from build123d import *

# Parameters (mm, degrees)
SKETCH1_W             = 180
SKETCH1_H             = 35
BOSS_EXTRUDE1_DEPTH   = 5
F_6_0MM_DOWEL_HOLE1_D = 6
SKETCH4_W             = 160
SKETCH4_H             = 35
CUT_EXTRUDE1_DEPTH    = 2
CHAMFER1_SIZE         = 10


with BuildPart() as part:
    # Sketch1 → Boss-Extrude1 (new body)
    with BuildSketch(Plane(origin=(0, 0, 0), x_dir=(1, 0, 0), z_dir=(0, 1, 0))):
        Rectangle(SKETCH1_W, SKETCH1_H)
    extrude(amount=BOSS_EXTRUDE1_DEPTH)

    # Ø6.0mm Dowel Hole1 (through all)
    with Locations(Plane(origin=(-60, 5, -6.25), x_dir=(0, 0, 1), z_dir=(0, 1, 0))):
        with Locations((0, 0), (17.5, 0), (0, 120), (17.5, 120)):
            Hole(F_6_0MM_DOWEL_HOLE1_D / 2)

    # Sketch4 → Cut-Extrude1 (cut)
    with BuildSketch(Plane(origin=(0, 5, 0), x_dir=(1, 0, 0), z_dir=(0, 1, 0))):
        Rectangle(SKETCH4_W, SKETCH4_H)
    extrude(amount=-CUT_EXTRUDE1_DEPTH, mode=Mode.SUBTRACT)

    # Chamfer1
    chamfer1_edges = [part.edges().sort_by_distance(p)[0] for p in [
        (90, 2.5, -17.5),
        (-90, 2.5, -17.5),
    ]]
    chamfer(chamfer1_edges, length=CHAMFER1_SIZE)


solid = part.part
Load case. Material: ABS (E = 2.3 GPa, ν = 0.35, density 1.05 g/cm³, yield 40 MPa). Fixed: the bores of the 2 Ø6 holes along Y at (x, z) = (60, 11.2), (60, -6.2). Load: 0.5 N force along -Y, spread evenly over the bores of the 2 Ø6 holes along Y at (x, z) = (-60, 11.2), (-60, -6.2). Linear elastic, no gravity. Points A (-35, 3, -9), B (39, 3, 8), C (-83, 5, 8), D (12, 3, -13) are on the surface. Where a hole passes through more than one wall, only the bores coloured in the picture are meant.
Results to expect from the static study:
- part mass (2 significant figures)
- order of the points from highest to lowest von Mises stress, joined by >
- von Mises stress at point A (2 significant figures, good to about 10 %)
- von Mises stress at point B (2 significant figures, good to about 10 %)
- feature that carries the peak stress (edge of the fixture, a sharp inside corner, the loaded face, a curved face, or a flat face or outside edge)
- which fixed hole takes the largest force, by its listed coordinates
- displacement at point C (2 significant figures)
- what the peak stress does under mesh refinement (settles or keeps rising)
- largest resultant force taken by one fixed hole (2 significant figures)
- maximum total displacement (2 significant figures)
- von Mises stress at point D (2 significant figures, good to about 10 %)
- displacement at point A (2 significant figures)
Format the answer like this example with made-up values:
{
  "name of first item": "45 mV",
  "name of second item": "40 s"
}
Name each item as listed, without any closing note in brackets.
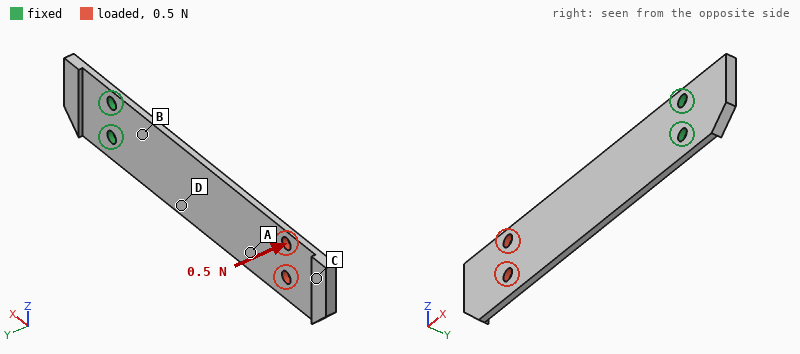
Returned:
{
  "part mass": "20 g",
  "order of the points from highest to lowest von Mises stress, joined by >": "B > D > A > C",
  "von Mises stress at point A": "0.24 MPa",
  "von Mises stress at point B": "0.90 MPa",
  "feature that carries the peak stress": "edge of the fixture",
  "which fixed hole takes the largest force, by its listed coordinates": "(60, -6.2)",
  "displacement at point C": "1.9 mm",
  "what the peak stress does under mesh refinement": "keeps rising",
  "largest resultant force taken by one fixed hole": "0.34 N",
  "maximum total displacement": "2.1 mm",
  "von Mises stress at point D": "0.69 MPa",
  "displacement at point A": "1.0 mm"
}
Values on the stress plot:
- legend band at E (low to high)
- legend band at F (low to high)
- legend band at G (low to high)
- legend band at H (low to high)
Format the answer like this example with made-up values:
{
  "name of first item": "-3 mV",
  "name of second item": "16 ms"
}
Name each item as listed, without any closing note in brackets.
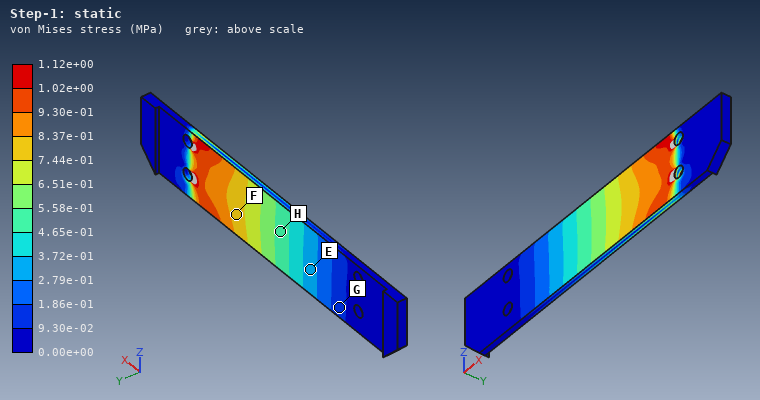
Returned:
{
  "legend band at E": "2.79e-01 to 3.72e-01 MPa",
  "legend band at F": "7.44e-01 to 8.37e-01 MPa",
  "legend band at G": "9.30e-02 to 1.86e-01 MPa",
  "legend band at H": "4.65e-01 to 5.58e-01 MPa"
}
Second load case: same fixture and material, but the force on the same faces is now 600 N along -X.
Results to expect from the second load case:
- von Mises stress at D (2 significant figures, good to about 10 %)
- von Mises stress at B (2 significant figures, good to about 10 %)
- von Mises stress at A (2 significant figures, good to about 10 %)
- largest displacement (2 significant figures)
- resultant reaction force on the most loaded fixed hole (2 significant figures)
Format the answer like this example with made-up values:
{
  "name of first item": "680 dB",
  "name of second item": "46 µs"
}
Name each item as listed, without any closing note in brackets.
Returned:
{
  "von Mises stress at D": "3.9 MPa",
  "von Mises stress at B": "6.9 MPa",
  "von Mises stress at A": "4.5 MPa",
  "largest displacement": "0.75 mm",
  "resultant reaction force on the most loaded fixed hole": "310 N"
}
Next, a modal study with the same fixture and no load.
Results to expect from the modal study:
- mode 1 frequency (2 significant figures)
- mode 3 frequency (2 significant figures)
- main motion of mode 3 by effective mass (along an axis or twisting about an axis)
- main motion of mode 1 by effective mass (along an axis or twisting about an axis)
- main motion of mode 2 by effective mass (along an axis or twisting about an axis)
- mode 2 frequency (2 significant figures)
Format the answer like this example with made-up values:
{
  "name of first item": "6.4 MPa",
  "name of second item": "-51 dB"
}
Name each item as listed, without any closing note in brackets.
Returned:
{
  "mode 1 frequency": "32 Hz",
  "mode 3 frequency": "270 Hz",
  "main motion of mode 3 by effective mass": "twisting about X",
  "main motion of mode 1 by effective mass": "along Y",
  "main motion of mode 2 by effective mass": "along Y",
  "mode 2 frequency": "200 Hz"
}
